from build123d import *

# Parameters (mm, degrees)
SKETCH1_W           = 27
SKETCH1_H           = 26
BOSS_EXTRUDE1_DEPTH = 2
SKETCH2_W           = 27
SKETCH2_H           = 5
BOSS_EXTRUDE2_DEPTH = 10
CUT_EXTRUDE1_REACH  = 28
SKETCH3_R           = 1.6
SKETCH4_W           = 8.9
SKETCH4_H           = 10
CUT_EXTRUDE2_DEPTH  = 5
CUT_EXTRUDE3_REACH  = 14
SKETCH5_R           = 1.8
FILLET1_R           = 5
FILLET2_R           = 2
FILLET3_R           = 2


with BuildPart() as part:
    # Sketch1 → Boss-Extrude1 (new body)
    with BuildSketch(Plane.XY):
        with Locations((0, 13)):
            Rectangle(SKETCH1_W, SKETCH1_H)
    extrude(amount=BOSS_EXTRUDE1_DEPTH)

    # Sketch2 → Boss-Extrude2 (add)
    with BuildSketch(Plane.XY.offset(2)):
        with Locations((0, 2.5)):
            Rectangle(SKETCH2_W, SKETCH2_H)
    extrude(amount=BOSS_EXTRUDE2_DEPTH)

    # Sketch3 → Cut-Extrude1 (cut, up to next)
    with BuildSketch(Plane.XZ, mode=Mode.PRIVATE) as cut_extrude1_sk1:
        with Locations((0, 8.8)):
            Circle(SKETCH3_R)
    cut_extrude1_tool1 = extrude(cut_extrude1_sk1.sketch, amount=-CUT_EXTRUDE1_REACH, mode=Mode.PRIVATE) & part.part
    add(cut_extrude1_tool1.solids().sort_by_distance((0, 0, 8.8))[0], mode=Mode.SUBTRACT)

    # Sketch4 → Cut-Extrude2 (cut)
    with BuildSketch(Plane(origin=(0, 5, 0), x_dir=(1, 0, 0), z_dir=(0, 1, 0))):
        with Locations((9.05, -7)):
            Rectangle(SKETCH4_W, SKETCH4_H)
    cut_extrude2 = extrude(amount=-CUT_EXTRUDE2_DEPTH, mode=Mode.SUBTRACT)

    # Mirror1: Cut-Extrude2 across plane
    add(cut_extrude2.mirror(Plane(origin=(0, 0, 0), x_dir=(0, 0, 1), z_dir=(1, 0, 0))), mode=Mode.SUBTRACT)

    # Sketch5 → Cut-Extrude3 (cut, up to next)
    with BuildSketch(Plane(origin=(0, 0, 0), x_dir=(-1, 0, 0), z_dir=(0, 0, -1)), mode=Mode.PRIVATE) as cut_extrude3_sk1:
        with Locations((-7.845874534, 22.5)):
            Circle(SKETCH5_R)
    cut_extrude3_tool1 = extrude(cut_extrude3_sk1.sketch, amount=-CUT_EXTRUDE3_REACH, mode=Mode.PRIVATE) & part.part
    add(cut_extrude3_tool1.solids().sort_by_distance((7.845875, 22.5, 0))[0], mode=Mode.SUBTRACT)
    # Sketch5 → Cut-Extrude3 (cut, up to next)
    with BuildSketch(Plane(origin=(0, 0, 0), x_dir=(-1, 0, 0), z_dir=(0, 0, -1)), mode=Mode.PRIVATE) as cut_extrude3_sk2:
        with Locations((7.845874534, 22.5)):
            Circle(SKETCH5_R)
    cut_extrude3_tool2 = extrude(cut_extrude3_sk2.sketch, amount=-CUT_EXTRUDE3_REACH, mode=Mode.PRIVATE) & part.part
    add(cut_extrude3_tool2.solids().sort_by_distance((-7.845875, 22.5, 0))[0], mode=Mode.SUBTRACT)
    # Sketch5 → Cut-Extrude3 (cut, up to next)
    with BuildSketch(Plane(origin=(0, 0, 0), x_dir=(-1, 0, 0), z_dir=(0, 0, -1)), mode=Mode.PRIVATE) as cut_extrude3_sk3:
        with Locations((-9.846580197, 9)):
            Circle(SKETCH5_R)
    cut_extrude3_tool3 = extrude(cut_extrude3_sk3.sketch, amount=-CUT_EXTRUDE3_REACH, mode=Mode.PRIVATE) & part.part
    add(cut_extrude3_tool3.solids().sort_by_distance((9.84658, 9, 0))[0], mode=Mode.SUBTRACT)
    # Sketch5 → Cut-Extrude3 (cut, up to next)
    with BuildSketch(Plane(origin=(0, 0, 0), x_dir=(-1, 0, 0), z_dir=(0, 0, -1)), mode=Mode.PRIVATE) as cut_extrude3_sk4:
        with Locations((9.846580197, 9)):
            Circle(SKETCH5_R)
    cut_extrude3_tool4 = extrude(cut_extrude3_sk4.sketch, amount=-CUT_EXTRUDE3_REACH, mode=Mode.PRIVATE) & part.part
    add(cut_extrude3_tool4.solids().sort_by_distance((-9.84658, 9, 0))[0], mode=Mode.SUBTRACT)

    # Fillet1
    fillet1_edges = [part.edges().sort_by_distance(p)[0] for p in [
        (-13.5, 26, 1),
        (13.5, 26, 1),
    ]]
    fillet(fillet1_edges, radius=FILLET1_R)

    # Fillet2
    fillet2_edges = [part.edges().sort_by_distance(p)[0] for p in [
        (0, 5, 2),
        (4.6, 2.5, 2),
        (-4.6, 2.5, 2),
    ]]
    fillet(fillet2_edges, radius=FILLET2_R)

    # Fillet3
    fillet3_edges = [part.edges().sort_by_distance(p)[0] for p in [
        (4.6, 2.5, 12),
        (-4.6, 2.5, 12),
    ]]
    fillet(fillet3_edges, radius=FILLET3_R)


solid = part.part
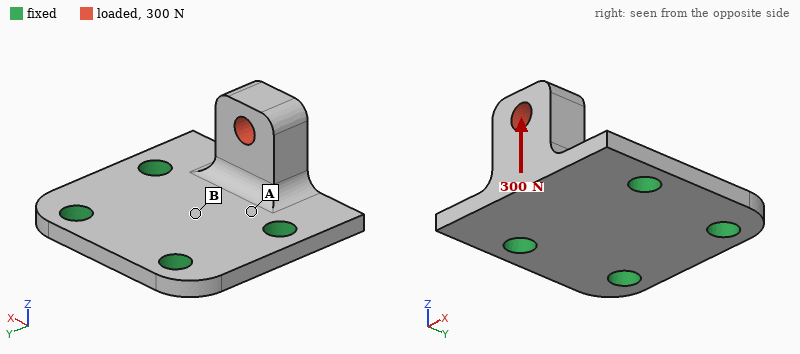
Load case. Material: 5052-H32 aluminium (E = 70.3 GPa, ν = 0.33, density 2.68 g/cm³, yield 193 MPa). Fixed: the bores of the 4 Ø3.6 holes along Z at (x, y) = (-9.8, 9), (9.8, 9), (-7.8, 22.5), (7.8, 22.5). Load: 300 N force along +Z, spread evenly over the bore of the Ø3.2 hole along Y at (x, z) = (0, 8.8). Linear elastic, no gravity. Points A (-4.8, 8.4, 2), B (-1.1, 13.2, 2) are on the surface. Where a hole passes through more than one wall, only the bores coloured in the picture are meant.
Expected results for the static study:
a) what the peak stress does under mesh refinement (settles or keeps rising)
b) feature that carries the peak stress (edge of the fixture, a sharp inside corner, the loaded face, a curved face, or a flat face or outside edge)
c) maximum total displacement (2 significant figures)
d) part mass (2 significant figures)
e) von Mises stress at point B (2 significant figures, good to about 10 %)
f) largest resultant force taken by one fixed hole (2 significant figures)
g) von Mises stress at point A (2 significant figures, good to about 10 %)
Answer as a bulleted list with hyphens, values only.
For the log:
- keeps rising
- edge of the fixture
- 65 µm
- 4.6 g
- 19 MPa
- 170 N
- 51 MPa
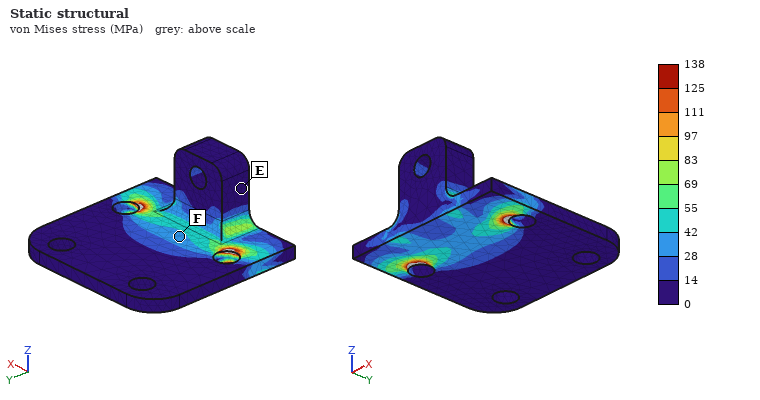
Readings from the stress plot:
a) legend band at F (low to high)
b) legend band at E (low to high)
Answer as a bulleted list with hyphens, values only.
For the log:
- 28 to 42 MPa
- 0 to 14 MPa
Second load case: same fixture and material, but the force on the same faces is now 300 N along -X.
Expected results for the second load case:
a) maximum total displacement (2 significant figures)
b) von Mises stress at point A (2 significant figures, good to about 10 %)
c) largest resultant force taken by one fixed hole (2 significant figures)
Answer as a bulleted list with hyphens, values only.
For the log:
- 25 µm
- 25 MPa
- 230 N
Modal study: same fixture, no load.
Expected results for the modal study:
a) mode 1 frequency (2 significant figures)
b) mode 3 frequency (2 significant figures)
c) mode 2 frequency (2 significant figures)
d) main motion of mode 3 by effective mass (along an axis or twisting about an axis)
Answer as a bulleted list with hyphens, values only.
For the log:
- 9000 Hz
- 24 kHz
- 21 kHz
- along Z
